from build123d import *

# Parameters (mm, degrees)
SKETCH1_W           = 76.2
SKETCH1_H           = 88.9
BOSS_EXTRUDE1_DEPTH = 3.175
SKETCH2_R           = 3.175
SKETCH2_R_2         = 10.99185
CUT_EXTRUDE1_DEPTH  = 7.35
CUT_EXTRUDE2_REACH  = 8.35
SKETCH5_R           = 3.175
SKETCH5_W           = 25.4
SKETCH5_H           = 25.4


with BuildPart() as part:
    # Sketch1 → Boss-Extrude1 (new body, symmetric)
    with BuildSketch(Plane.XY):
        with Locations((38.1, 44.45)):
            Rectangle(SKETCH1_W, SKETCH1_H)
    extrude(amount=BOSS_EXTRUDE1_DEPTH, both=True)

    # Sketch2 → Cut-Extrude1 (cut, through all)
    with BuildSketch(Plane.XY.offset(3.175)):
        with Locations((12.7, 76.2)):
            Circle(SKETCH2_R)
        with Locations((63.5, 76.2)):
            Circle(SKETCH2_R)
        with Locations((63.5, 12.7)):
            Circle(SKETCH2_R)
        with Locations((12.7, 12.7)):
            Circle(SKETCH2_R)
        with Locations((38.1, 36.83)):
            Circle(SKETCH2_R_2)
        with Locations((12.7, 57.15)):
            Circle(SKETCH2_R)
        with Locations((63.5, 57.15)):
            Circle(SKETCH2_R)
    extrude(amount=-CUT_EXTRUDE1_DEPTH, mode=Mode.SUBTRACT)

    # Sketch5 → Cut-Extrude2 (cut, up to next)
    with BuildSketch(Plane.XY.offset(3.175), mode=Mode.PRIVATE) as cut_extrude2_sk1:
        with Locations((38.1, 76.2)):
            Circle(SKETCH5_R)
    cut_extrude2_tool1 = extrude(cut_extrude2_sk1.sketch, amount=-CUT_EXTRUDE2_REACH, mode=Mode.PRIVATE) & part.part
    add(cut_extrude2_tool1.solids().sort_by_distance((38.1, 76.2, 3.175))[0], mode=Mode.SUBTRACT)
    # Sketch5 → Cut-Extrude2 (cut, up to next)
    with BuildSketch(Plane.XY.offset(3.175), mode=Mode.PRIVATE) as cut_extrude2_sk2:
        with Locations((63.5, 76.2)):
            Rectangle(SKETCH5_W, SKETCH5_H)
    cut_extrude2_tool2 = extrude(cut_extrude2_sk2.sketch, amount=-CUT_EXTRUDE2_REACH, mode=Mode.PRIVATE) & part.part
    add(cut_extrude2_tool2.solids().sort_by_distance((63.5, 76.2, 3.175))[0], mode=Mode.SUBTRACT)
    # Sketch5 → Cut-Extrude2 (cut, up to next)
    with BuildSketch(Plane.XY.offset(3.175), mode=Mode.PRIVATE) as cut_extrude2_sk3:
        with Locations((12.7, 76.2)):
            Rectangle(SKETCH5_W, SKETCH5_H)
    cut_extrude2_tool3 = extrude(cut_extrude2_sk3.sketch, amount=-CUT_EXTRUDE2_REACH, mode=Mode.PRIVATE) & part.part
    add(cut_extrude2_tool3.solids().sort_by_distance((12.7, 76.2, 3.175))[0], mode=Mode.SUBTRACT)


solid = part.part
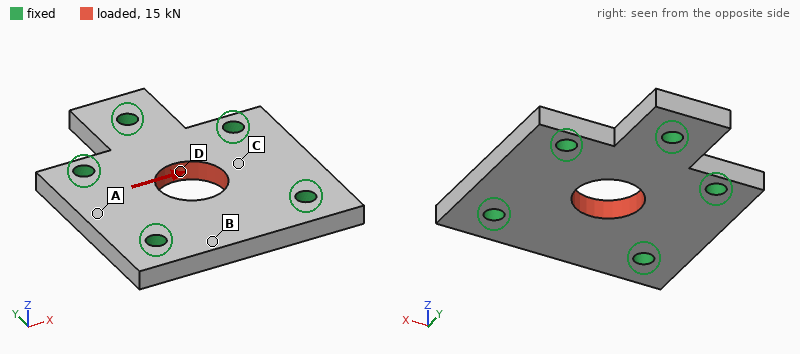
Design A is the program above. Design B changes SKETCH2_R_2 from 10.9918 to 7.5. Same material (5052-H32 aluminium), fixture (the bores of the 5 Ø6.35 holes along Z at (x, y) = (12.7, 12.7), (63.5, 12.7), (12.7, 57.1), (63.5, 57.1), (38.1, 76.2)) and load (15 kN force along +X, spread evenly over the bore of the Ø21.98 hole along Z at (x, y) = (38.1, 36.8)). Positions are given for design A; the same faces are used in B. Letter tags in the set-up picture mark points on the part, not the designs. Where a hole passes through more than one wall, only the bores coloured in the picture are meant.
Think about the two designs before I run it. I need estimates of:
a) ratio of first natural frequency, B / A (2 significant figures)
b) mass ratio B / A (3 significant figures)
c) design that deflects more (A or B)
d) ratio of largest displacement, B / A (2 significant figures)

0.94
1.04
B
1.2
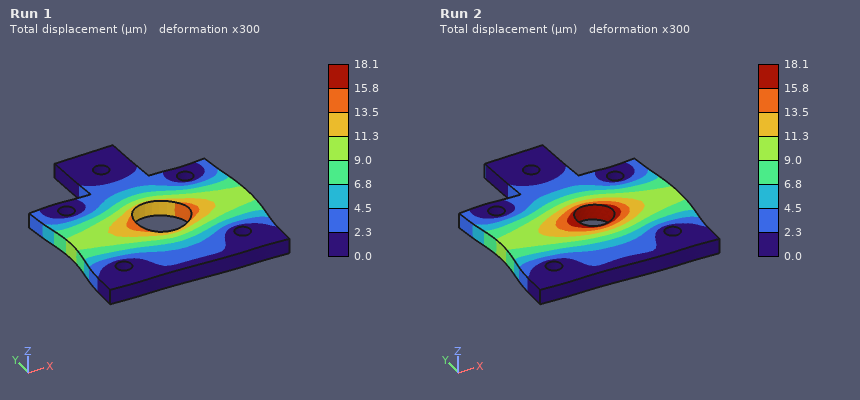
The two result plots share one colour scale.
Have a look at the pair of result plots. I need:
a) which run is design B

Run 2
